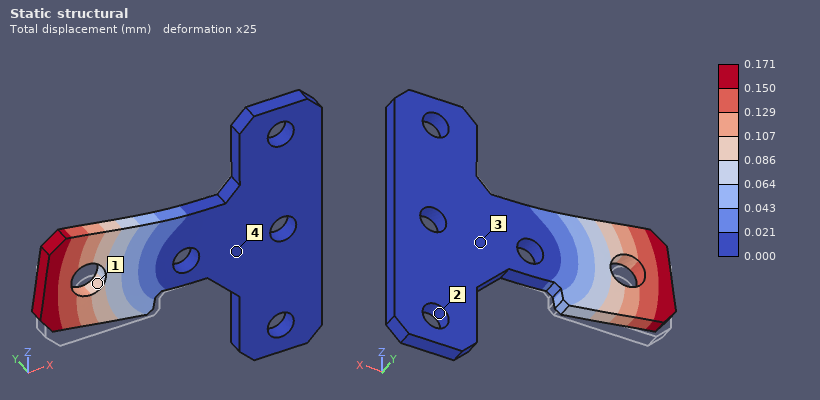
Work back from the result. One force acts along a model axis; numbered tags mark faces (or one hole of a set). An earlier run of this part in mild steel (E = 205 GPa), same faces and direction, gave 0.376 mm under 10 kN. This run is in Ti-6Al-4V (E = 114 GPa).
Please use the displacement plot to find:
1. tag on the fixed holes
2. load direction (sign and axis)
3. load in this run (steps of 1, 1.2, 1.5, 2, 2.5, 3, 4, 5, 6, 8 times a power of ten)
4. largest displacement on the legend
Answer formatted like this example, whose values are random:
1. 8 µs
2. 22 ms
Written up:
1. 2
2. +Z
3. 2.5 kN
4. 0.171 mm
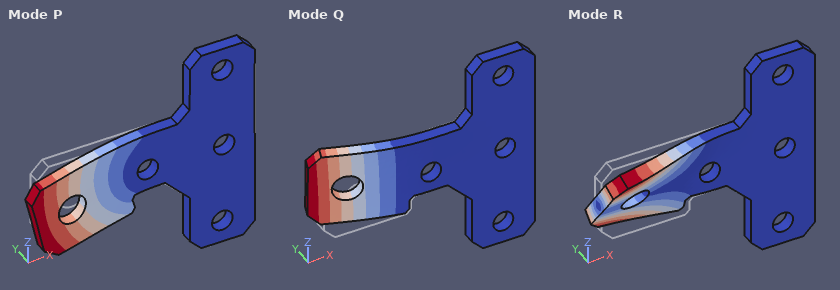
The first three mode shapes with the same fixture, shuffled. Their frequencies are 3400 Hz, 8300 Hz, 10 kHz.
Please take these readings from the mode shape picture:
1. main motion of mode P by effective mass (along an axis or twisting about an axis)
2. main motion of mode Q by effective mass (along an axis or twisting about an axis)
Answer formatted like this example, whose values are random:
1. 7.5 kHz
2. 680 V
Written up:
1. along Z
2. along Y
